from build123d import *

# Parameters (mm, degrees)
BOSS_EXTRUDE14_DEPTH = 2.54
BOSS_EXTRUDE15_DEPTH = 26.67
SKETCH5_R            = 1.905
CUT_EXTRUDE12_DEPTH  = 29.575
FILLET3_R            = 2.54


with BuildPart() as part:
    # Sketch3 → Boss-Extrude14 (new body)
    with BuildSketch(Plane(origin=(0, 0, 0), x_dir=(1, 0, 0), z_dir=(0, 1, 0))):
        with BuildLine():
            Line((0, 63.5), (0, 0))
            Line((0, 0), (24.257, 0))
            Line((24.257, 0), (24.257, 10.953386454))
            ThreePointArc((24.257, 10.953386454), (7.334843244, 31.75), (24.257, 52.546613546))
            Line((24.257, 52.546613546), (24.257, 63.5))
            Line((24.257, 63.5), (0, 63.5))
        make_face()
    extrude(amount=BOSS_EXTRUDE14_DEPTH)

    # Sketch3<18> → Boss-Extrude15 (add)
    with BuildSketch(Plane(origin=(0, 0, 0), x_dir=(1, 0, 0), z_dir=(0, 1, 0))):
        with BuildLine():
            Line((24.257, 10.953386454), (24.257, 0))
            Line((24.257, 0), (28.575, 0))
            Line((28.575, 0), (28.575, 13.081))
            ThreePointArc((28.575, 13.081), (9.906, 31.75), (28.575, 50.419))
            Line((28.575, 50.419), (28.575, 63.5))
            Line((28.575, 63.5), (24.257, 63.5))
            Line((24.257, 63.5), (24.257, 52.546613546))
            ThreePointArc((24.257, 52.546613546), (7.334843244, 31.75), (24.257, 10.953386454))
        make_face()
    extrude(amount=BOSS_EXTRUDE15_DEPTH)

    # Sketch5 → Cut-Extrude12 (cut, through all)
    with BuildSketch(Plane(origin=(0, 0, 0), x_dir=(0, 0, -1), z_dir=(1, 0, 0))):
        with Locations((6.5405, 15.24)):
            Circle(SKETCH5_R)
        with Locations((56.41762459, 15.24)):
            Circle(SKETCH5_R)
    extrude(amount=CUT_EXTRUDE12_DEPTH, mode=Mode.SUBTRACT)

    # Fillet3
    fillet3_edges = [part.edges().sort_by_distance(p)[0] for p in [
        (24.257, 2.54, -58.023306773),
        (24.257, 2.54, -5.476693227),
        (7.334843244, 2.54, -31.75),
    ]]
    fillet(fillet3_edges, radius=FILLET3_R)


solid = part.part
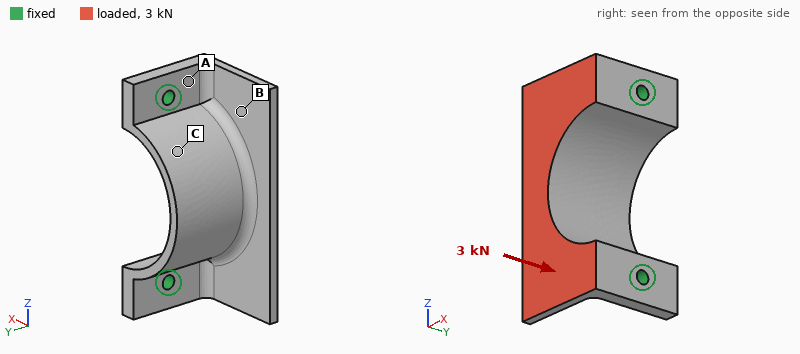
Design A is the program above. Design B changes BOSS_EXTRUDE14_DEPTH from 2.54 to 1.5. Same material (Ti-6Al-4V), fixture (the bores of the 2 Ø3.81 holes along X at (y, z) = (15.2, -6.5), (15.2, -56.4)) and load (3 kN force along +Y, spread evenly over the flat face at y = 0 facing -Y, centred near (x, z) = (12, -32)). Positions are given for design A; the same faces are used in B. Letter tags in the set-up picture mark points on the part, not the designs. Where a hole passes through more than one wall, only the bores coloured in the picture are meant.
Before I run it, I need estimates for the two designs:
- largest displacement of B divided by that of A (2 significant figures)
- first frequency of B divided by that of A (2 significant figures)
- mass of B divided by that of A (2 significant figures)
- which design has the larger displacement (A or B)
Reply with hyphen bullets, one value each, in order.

- 2.4
- 1.0
- 0.89
- B
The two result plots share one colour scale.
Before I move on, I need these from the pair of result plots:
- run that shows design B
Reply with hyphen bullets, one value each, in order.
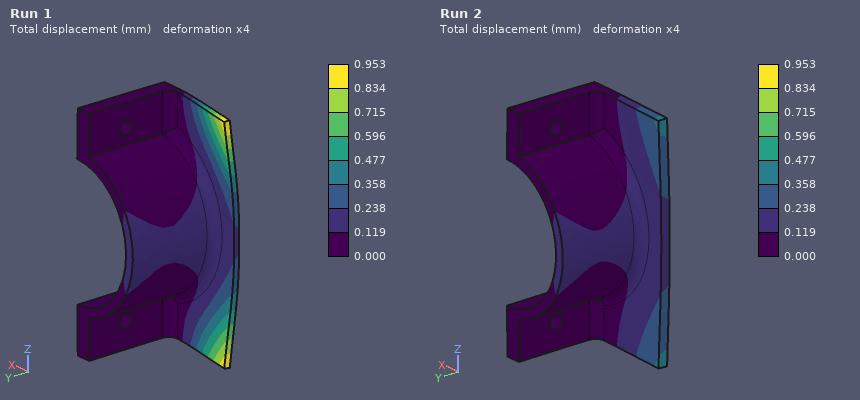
- Run 1
